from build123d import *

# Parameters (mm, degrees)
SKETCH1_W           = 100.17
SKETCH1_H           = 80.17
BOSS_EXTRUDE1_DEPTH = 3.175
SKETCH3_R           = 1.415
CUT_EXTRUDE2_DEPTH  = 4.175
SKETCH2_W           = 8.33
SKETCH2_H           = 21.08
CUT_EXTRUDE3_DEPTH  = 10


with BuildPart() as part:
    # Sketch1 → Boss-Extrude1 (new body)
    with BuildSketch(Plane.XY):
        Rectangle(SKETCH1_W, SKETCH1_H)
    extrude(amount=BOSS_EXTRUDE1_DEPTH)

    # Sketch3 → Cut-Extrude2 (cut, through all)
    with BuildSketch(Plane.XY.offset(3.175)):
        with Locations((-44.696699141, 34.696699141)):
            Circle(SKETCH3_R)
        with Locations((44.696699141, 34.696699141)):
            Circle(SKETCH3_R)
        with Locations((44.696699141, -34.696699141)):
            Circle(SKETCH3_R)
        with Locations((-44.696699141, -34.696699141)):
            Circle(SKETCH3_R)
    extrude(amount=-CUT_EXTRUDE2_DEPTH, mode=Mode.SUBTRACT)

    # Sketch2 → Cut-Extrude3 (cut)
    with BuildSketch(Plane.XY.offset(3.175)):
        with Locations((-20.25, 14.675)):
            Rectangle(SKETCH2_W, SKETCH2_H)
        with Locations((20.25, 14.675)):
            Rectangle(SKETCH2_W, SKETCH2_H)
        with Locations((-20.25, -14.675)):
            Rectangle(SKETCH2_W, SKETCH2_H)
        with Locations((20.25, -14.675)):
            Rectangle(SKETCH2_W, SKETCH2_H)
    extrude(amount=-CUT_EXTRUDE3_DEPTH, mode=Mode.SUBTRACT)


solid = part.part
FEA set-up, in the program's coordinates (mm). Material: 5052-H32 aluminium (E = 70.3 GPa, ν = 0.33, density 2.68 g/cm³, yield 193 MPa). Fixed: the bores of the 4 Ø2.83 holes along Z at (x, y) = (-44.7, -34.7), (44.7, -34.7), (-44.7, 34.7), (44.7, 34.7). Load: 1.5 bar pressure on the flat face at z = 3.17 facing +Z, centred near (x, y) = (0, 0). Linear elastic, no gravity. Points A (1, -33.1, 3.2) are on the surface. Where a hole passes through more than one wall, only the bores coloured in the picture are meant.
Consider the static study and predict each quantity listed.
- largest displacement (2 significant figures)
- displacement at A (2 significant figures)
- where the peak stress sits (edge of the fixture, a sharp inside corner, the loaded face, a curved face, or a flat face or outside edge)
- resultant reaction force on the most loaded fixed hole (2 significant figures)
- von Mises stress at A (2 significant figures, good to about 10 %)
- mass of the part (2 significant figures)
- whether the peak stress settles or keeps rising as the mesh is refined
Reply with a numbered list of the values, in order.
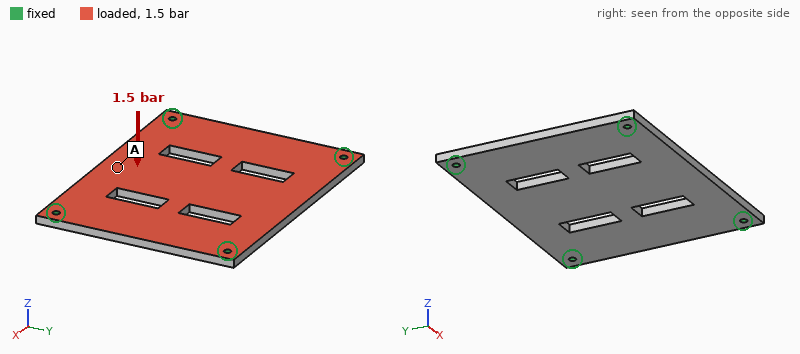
1. 0.28 mm
2. 0.22 mm
3. edge of the fixture
4. 270 N
5. 36 MPa
6. 62 g
7. keeps rising
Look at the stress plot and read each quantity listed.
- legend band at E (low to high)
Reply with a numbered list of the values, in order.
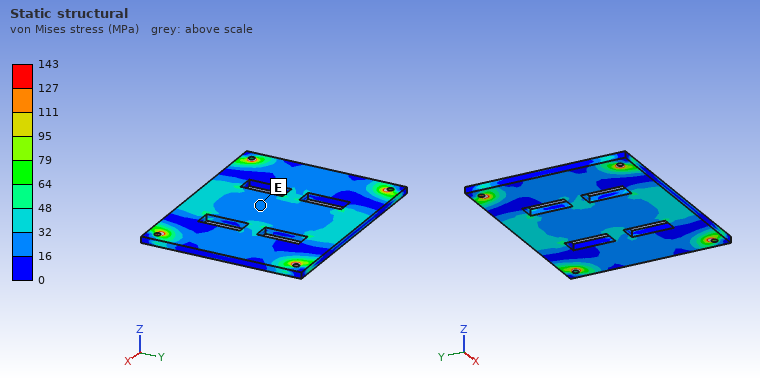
1. 16 to 32 MPa
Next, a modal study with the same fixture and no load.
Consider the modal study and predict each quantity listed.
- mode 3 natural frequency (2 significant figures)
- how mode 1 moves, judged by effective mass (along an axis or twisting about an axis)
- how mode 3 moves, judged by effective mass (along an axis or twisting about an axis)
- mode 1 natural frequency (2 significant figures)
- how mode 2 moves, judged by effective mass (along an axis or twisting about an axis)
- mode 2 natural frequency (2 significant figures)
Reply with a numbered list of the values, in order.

1. 3100 Hz
2. along Z
3. twisting about Y
4. 1500 Hz
5. twisting about X
6. 2400 Hz
